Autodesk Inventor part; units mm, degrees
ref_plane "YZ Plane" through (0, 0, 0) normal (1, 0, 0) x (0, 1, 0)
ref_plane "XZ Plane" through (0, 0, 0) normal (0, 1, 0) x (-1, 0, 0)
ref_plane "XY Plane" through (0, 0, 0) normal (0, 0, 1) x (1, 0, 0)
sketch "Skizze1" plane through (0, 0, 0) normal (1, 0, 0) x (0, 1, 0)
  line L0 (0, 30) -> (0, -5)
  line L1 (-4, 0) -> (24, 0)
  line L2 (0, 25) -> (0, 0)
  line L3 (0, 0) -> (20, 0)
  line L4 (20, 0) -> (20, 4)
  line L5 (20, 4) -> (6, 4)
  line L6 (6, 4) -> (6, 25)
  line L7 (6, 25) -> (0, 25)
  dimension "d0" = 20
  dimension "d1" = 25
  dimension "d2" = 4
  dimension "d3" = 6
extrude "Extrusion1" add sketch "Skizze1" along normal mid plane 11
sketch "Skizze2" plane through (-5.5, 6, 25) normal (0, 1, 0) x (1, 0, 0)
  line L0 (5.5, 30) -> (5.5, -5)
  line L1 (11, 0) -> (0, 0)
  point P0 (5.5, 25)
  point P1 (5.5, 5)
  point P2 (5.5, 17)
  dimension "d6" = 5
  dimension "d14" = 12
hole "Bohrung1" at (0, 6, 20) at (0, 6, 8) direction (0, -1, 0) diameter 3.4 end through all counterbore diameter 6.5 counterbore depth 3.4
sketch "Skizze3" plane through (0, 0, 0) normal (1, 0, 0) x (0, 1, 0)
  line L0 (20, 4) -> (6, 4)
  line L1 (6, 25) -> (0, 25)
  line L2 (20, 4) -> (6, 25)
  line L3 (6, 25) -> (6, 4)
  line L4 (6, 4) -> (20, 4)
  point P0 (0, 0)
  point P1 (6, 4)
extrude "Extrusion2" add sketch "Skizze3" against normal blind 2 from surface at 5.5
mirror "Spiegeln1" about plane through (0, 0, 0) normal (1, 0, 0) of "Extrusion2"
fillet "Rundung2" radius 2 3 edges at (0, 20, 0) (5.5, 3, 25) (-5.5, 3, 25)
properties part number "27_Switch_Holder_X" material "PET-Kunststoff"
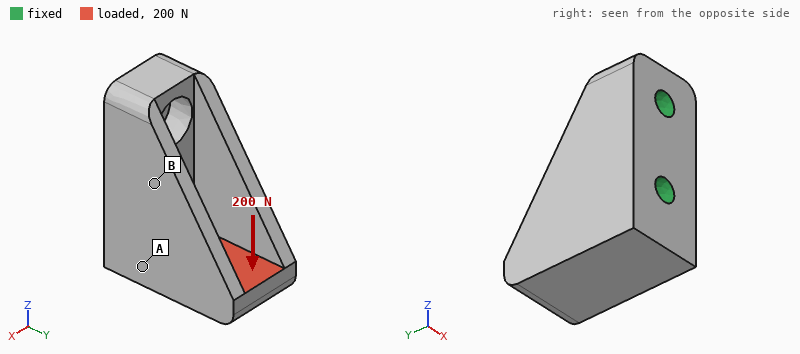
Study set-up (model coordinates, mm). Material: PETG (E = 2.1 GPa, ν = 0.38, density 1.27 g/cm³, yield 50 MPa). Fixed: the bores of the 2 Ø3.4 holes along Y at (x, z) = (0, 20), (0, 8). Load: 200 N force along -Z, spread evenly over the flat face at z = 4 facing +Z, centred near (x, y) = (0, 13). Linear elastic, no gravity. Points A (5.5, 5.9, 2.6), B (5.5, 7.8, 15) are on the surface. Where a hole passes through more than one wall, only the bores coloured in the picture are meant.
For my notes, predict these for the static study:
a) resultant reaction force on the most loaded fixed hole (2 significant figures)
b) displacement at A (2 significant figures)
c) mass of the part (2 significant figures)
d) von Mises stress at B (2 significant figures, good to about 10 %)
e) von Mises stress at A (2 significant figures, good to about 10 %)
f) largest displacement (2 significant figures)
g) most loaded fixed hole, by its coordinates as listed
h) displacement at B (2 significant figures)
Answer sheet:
210 N
0.074 mm
3.3 g
6.1 MPa
2.3 MPa
0.21 mm
(0, 20)
0.046 mm
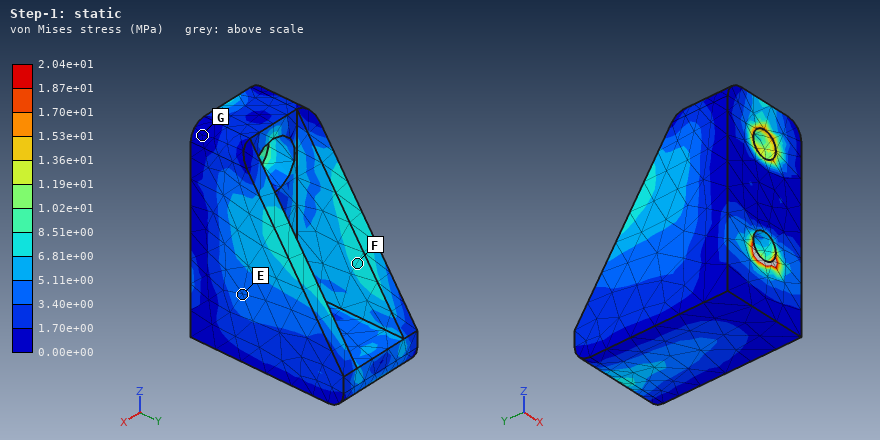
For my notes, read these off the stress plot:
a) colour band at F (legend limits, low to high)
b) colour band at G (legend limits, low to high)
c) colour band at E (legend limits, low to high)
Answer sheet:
6.81e+00 to 8.51e+00 MPa
0.00e+00 to 1.70e+00 MPa
3.40e+00 to 5.11e+00 MPa
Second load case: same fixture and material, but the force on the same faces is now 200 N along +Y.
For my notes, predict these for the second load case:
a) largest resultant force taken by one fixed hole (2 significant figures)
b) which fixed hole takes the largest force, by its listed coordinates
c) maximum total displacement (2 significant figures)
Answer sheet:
240 N
(0, 8)
0.10 mm
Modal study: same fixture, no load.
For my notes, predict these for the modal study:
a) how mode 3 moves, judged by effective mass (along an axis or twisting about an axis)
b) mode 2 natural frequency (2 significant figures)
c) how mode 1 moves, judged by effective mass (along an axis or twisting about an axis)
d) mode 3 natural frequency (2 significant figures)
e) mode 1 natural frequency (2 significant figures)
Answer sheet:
twisting about Y
4800 Hz
along X
7600 Hz
2400 Hz
